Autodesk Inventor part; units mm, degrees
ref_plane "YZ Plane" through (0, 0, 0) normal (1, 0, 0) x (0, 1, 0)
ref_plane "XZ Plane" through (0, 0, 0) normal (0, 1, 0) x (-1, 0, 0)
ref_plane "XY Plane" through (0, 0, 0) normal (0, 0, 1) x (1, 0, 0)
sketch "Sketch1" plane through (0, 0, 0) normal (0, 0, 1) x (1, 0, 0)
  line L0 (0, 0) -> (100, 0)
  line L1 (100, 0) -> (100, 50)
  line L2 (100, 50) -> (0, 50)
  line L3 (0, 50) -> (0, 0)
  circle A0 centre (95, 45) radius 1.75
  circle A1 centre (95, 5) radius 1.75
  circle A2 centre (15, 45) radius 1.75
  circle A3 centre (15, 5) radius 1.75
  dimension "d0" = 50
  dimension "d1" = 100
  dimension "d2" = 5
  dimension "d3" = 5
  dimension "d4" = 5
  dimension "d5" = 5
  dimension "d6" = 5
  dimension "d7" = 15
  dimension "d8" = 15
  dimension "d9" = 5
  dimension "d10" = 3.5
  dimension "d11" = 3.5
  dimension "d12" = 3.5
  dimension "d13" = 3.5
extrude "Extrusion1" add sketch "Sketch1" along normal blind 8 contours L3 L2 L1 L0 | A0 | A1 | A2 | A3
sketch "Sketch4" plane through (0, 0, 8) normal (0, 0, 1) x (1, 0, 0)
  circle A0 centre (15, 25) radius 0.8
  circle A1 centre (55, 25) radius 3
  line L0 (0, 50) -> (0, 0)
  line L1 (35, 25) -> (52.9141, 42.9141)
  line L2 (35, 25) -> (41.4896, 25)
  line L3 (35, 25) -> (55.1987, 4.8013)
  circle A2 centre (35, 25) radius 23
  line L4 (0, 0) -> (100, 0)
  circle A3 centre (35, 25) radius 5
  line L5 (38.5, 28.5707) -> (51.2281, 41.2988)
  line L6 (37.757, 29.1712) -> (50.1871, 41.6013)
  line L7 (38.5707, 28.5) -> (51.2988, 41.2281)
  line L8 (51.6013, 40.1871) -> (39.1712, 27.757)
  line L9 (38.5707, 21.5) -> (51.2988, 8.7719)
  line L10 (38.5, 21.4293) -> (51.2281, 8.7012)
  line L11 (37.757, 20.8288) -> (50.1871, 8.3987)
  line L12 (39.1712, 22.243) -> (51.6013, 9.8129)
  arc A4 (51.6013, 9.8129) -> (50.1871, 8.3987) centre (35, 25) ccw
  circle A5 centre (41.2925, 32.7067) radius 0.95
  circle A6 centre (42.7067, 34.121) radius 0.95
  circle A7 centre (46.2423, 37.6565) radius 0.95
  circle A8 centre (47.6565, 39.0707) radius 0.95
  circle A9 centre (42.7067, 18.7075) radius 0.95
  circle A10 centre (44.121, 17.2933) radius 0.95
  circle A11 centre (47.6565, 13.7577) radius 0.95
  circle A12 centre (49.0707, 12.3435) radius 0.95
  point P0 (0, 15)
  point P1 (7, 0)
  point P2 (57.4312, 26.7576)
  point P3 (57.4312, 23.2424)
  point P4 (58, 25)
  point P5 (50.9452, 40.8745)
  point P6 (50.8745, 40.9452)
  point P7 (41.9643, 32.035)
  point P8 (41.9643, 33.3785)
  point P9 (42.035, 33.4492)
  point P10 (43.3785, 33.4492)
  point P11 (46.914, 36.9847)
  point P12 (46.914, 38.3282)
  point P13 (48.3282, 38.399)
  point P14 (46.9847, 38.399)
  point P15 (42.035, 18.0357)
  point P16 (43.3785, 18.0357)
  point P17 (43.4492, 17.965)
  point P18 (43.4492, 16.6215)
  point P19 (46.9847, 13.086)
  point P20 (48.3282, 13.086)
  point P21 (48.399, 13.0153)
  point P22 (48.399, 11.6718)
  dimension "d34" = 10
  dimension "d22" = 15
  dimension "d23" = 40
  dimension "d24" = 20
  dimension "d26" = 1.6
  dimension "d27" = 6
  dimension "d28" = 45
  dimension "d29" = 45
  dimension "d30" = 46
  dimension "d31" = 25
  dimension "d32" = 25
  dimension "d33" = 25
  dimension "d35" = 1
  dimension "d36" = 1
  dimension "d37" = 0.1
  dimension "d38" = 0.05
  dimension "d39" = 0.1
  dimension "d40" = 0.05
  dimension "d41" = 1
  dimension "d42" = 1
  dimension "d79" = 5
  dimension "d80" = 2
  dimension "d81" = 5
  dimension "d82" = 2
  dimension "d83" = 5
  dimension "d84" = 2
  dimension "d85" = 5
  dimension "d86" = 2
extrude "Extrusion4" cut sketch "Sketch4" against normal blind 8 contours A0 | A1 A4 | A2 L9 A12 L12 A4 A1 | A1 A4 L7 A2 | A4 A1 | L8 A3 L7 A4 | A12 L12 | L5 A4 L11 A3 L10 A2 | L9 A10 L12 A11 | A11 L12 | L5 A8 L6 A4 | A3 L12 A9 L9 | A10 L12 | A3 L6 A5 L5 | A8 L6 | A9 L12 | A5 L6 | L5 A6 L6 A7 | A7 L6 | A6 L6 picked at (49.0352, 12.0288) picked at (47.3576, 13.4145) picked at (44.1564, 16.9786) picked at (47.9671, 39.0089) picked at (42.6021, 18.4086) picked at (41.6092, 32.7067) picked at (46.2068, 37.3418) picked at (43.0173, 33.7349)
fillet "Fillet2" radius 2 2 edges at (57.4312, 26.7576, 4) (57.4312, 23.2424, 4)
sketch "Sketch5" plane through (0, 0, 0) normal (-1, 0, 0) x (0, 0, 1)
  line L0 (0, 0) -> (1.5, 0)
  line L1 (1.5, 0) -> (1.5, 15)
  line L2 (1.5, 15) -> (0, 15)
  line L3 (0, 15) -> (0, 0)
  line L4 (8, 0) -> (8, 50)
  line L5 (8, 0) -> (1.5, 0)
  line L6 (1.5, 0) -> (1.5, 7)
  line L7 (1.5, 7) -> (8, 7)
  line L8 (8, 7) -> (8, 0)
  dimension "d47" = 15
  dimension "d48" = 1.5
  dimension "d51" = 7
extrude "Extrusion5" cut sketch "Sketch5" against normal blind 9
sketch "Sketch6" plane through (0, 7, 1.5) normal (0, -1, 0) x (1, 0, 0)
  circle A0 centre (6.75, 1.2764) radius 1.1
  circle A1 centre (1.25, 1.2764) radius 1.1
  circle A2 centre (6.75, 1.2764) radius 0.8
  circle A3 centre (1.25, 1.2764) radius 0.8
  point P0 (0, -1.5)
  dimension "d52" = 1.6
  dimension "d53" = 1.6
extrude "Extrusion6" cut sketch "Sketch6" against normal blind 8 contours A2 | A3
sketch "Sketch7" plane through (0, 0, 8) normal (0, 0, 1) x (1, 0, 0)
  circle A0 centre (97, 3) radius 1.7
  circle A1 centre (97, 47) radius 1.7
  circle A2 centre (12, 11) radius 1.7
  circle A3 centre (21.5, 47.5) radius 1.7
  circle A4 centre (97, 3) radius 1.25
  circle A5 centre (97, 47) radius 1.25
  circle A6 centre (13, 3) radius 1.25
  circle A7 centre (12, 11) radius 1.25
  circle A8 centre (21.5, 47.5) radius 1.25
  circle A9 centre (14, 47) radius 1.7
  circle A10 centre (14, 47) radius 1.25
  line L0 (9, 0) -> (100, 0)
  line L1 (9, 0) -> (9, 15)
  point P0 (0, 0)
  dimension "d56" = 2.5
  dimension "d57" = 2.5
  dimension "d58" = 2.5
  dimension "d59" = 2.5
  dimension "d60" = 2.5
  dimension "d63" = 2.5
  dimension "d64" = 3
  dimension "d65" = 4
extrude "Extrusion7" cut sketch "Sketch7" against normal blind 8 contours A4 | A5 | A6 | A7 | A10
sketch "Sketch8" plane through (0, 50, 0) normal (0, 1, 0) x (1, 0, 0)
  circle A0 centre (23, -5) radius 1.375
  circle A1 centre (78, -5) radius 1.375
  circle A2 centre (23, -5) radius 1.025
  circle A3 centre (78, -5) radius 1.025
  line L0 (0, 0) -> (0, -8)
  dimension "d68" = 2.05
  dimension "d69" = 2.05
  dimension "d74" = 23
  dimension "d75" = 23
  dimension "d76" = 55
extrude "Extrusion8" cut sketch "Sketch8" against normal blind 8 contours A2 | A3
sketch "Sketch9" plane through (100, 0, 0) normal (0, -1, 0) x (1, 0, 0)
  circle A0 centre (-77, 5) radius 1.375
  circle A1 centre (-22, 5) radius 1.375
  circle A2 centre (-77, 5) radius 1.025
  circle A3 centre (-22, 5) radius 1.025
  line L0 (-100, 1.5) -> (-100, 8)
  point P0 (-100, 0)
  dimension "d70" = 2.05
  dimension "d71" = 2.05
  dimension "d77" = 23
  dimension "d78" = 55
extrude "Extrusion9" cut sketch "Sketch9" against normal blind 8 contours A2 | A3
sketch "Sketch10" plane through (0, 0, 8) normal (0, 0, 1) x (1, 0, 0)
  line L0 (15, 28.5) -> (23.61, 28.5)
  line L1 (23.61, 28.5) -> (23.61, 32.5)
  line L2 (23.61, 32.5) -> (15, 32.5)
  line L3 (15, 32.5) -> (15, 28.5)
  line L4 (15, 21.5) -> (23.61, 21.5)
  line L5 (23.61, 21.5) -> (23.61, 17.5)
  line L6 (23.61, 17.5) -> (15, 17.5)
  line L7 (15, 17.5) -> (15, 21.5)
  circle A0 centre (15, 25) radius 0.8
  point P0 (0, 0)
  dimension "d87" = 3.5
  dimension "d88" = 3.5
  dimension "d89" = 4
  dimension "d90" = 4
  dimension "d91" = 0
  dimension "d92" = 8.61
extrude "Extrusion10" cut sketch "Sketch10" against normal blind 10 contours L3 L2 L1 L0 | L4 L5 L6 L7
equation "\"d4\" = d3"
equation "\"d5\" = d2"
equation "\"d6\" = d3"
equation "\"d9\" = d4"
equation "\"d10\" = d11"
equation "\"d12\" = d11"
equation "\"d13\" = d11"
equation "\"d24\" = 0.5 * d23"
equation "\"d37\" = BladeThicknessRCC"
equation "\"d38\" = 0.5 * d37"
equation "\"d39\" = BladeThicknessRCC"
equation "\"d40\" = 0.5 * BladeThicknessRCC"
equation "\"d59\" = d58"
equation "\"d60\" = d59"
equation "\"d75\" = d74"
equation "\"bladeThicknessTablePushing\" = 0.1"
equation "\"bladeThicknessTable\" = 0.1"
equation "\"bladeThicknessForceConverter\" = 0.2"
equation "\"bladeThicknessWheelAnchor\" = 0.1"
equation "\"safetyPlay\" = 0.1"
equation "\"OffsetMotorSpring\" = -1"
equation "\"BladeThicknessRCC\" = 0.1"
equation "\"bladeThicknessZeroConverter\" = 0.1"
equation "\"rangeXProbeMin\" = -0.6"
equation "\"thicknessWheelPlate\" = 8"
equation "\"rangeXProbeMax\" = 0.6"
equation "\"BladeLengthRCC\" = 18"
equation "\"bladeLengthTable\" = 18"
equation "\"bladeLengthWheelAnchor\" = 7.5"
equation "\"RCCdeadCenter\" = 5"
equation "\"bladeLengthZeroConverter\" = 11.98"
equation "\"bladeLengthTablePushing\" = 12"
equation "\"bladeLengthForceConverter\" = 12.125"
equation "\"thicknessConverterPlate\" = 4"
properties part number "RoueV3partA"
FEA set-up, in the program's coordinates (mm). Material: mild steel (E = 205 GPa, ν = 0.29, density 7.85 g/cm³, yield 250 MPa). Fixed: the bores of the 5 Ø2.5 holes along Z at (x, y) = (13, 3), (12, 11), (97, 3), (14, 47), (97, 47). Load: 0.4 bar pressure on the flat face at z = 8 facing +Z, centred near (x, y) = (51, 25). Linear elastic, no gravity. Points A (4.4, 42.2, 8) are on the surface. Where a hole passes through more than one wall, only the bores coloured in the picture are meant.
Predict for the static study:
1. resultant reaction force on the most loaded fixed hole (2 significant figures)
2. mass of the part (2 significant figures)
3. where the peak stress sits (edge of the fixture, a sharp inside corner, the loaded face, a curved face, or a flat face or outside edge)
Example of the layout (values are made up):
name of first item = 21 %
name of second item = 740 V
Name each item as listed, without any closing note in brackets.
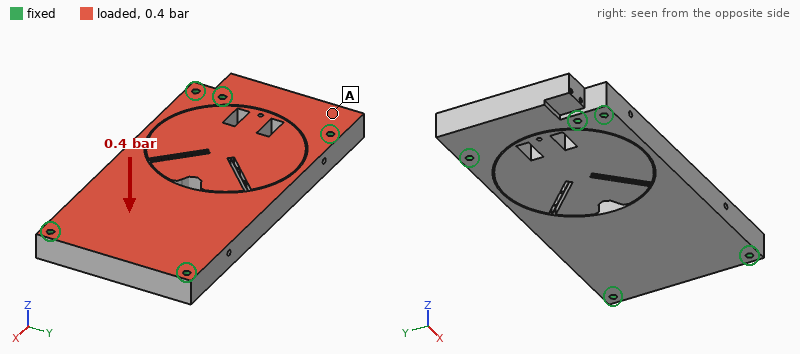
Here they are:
resultant reaction force on the most loaded fixed hole = 50 N
mass of the part = 290 g
where the peak stress sits = a flat face or outside edge
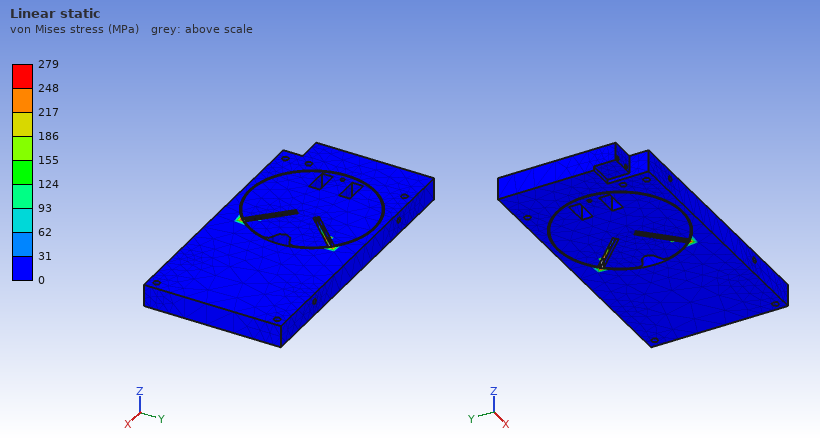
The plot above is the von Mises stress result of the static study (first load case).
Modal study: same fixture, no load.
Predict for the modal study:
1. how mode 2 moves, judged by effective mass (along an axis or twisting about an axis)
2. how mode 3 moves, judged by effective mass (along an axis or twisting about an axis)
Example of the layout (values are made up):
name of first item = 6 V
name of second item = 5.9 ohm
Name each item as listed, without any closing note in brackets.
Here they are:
how mode 2 moves, judged by effective mass = along Z
how mode 3 moves, judged by effective mass = along Y
